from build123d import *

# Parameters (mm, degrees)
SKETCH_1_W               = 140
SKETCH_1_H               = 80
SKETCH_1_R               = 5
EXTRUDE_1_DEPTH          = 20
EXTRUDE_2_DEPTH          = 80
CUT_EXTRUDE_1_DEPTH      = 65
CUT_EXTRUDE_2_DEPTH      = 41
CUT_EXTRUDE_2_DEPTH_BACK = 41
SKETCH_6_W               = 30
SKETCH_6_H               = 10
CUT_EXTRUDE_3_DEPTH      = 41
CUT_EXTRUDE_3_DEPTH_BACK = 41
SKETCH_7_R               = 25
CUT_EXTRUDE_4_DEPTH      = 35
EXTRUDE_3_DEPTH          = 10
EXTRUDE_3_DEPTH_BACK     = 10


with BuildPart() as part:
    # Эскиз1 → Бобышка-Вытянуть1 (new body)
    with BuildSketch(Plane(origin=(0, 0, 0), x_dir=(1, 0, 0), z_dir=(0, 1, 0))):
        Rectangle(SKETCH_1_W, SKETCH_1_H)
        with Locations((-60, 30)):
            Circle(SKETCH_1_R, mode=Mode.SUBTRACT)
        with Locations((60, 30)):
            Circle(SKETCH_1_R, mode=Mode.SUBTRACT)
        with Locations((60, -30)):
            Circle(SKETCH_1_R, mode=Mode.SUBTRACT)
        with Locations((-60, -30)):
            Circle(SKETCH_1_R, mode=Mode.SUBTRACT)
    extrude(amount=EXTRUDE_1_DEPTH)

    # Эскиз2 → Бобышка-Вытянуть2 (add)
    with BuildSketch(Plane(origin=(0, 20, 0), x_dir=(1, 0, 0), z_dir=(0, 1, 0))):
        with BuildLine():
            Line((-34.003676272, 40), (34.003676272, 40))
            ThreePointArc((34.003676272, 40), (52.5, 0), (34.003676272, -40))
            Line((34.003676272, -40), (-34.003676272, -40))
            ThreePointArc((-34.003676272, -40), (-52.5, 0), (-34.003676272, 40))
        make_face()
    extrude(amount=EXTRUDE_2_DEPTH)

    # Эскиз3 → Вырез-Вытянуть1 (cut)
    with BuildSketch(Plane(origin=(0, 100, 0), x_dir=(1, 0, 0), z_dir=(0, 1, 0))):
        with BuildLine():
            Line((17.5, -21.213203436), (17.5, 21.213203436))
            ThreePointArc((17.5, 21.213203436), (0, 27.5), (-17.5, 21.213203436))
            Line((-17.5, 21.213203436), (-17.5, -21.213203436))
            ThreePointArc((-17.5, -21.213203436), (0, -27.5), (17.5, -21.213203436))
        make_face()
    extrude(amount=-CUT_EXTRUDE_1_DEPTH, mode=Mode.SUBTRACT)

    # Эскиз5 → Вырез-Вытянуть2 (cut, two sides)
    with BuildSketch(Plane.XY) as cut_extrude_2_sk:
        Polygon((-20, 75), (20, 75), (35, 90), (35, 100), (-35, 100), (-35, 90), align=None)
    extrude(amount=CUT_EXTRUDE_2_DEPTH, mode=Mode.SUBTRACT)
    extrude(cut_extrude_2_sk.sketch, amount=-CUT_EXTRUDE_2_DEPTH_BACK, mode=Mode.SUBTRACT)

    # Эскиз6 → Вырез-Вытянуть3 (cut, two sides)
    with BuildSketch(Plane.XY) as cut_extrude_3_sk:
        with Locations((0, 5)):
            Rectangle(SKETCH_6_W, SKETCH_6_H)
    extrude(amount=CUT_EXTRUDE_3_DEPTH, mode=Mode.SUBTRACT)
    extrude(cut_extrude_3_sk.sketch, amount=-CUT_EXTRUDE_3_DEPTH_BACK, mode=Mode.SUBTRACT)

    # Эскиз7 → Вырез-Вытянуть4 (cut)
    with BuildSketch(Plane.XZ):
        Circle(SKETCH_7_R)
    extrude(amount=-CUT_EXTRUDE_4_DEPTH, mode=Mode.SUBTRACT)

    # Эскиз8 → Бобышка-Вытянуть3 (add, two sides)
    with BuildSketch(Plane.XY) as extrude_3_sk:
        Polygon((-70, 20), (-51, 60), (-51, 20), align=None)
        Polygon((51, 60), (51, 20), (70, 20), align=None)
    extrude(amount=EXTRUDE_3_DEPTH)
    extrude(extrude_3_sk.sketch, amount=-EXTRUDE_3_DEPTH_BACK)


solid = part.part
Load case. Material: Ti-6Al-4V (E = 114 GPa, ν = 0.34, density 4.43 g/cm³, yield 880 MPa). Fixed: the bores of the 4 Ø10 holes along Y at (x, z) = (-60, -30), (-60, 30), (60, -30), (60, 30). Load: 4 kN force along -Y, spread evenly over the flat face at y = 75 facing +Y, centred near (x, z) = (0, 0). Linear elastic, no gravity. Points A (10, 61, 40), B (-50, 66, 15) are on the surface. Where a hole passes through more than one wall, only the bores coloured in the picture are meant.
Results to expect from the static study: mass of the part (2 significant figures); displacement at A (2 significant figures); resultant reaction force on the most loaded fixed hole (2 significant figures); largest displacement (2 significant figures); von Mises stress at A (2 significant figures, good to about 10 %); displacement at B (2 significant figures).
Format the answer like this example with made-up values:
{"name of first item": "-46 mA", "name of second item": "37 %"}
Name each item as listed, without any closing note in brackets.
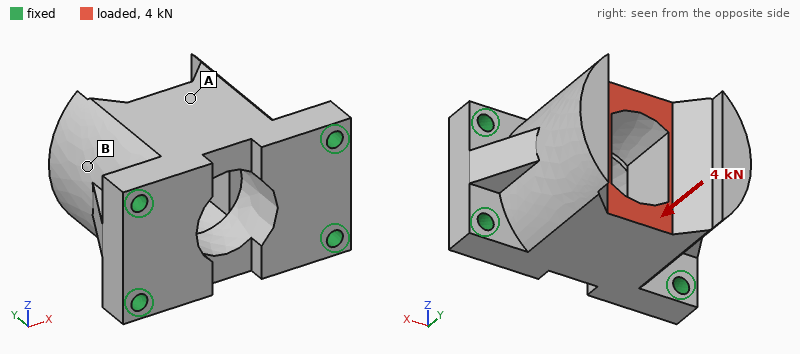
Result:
{"mass of the part": "2.5 kg", "displacement at A": "2.3 µm", "resultant reaction force on the most loaded fixed hole": "1.2 kN", "largest displacement": "2.8 µm", "von Mises stress at A": "2.4 MPa", "displacement at B": "1.2 µm"}
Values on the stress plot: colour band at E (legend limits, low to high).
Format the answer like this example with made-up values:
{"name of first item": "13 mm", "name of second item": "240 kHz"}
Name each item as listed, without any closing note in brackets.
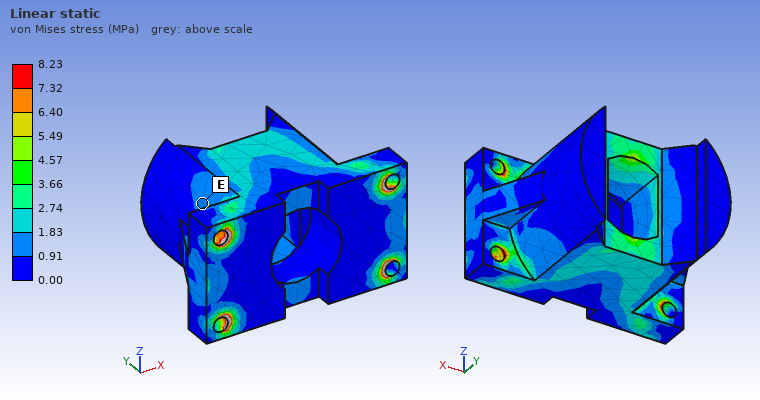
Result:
{"colour band at E": "0.91 to 1.83 MPa"}
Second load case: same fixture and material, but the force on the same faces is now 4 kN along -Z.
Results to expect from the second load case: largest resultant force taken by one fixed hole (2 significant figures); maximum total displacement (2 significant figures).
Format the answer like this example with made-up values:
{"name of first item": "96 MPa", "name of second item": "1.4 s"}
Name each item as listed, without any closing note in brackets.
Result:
{"largest resultant force taken by one fixed hole": "2.6 kN", "maximum total displacement": "13 µm"}
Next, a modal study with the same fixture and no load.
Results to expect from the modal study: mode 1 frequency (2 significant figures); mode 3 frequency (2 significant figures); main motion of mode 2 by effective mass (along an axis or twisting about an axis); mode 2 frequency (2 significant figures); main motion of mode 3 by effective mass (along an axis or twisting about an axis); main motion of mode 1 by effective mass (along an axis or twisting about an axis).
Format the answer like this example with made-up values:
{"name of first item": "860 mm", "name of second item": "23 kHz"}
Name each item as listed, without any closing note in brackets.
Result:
{"mode 1 frequency": "3200 Hz", "mode 3 frequency": "5700 Hz", "main motion of mode 2 by effective mass": "along X", "mode 2 frequency": "5300 Hz", "main motion of mode 3 by effective mass": "along Y", "main motion of mode 1 by effective mass": "along Z"}
